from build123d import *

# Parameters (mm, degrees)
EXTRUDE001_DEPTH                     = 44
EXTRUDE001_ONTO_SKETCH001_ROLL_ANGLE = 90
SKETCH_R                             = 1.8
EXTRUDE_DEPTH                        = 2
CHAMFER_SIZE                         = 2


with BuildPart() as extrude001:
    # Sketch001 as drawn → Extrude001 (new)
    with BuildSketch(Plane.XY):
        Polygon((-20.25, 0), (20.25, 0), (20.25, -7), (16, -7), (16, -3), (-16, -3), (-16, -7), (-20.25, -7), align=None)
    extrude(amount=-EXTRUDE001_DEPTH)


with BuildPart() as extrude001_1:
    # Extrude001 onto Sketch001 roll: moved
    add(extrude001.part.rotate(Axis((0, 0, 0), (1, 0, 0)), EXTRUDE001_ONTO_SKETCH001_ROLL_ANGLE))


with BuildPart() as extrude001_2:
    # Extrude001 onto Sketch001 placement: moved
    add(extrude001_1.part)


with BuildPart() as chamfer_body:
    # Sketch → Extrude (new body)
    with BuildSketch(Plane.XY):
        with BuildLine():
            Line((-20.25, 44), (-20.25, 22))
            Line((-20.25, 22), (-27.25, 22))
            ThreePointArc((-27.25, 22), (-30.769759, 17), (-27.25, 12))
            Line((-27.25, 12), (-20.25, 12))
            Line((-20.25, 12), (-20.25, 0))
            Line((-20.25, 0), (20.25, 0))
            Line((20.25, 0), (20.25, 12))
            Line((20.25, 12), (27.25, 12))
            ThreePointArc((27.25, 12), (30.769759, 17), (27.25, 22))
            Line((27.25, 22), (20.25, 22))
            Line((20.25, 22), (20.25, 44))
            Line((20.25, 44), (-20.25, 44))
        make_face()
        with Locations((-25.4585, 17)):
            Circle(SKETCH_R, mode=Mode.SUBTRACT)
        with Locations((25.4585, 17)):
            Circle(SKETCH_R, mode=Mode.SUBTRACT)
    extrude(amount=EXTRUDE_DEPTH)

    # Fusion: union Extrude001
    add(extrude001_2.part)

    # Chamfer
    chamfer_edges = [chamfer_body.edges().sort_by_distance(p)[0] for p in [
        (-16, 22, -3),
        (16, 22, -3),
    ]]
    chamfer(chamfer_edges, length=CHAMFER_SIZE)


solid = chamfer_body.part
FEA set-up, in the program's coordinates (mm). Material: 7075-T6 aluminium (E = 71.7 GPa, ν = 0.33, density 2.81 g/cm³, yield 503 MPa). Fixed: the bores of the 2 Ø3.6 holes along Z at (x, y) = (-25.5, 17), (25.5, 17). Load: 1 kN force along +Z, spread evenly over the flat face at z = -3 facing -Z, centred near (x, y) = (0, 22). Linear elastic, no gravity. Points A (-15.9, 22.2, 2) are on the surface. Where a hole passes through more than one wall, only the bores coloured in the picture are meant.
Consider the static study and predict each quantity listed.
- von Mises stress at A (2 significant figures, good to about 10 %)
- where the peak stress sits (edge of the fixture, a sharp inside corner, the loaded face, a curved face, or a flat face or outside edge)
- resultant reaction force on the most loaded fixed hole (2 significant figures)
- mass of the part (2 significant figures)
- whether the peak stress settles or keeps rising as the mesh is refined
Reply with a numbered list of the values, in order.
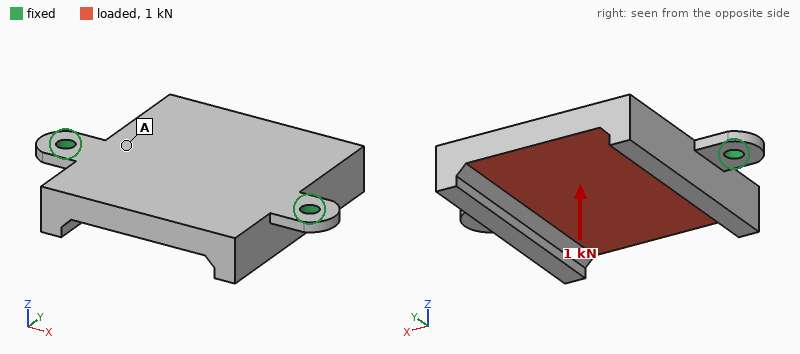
1. 32 MPa
2. edge of the fixture
3. 820 N
4. 31 g
5. keeps rising
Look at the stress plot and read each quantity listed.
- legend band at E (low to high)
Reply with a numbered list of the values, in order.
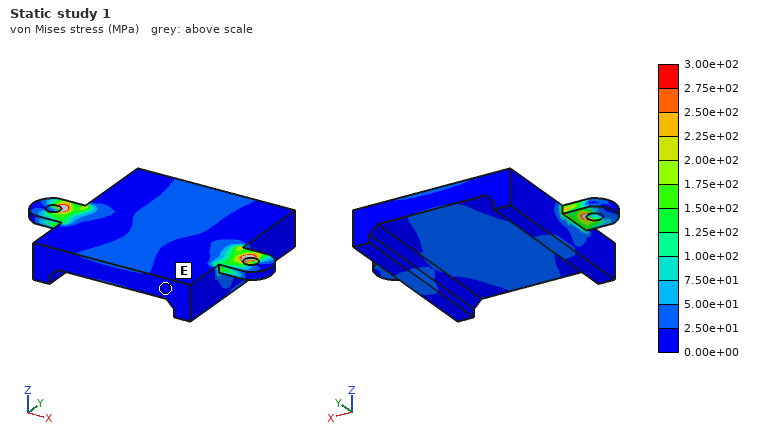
1. 0.00e+00 to 2.50e+01 MPa
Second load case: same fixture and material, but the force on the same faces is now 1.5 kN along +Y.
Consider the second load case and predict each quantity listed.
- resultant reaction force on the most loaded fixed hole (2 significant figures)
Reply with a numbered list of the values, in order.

1. 750 N
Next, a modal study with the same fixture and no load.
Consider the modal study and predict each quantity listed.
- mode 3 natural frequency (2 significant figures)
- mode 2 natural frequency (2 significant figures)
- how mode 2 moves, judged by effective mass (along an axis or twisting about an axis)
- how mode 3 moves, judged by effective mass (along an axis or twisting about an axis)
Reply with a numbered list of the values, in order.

1. 6900 Hz
2. 4900 Hz
3. along Z
4. twisting about Y
